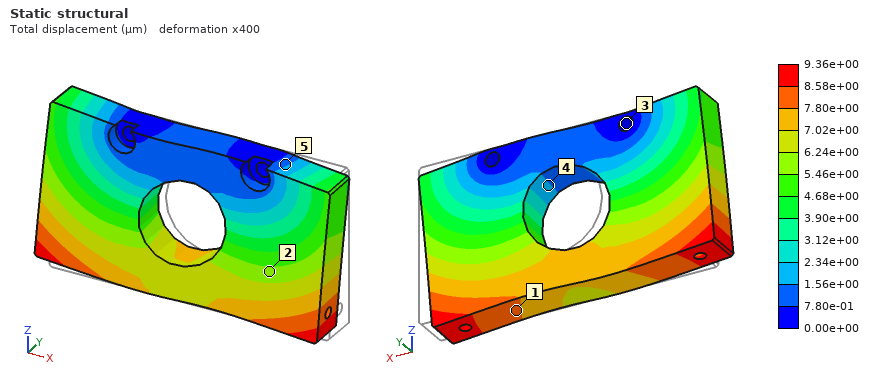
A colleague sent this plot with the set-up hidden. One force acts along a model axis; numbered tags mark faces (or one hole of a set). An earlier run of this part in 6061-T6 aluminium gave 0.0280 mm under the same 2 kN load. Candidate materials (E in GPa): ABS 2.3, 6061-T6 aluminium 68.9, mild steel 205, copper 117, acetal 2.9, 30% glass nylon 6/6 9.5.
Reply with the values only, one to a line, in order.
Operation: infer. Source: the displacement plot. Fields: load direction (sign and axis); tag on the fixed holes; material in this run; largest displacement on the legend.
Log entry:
-X
3
mild steel
9.36e+00 µm
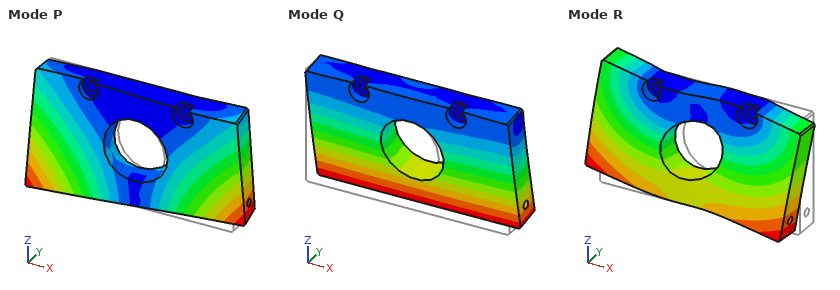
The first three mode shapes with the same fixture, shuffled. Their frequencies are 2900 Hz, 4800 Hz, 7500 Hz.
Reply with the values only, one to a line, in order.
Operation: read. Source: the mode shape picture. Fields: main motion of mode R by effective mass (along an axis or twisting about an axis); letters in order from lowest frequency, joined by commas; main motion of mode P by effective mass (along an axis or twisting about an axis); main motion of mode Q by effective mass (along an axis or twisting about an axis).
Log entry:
along X
Q, P, R
twisting about Z
along Y
